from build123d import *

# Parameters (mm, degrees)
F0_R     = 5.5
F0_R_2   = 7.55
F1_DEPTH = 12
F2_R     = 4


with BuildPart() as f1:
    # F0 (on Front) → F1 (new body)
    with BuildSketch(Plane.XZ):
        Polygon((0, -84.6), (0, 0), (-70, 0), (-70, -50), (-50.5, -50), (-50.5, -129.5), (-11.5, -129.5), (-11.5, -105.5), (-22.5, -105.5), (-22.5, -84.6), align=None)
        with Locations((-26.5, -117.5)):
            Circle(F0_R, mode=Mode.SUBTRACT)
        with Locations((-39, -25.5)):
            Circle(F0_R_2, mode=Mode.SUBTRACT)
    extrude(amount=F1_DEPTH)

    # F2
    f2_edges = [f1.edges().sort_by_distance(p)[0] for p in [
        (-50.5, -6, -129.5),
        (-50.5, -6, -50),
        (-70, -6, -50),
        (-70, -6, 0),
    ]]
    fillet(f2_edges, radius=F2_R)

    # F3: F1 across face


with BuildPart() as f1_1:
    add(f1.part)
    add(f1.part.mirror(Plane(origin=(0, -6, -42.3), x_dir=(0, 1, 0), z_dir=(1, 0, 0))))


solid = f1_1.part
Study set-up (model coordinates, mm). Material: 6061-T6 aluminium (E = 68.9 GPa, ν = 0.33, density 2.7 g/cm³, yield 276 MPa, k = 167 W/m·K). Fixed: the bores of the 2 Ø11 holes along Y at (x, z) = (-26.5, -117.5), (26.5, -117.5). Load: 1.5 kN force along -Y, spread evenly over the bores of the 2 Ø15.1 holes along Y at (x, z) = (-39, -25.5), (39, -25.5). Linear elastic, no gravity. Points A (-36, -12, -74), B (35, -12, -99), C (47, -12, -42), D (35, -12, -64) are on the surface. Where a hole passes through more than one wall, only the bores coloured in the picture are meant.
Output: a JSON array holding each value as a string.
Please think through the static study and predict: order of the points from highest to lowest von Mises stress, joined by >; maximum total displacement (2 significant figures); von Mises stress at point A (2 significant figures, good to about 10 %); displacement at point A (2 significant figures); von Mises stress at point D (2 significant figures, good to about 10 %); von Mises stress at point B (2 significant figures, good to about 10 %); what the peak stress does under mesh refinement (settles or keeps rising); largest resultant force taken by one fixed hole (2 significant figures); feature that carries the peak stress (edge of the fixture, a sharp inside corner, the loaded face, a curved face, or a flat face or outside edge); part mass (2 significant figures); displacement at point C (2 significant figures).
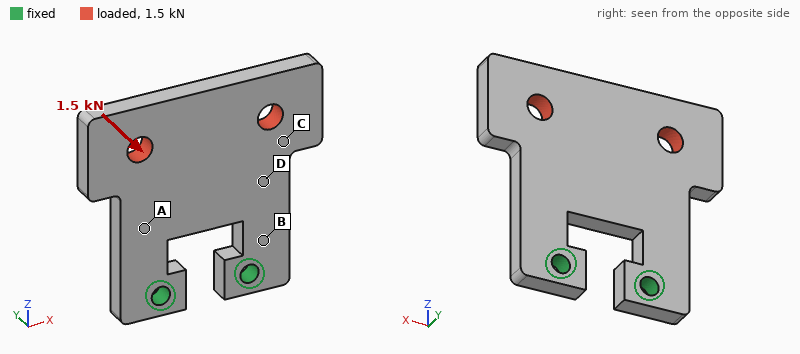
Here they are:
["B > A > D > C", "0.87 mm", "43 MPa", "0.19 mm", "28 MPa", "79 MPa", "keeps rising", "750 N", "edge of the fixture", "420 g", "0.46 mm"]
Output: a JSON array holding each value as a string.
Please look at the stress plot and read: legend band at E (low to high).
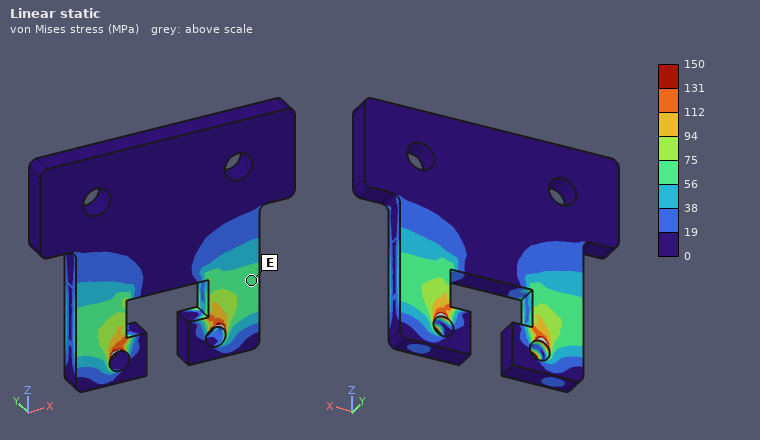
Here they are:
["56 to 75 MPa"]
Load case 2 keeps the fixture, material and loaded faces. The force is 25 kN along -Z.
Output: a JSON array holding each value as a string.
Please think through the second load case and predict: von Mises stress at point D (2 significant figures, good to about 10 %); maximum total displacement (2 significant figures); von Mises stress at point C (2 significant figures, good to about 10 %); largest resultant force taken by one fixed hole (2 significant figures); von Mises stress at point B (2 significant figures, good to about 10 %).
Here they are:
["30 MPa", "56 µm", "35 MPa", "13 kN", "40 MPa"]
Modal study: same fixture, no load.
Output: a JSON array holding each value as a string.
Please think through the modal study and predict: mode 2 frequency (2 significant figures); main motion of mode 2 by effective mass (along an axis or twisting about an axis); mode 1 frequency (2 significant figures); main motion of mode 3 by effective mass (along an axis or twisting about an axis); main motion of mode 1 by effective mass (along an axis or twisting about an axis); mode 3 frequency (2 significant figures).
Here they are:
["1200 Hz", "twisting about Z", "490 Hz", "along X", "along Y", "2200 Hz"]
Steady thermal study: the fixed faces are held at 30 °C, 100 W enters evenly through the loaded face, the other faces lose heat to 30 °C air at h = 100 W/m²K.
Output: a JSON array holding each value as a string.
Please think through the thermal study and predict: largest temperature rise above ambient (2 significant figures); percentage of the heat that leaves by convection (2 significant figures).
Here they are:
["32 K", "61 %"]
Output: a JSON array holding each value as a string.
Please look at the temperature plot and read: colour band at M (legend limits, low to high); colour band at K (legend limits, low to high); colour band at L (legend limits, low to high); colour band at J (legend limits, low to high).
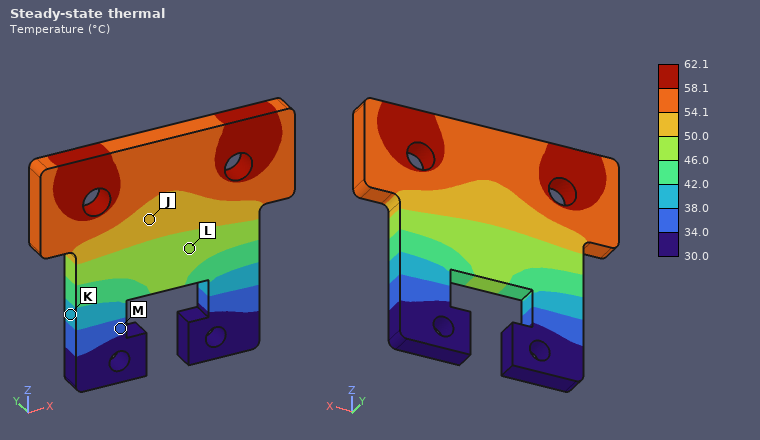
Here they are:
["34.0 to 38.0 °C", "38.0 to 42.0 °C", "46.0 to 50.0 °C", "50.0 to 54.1 °C"]
